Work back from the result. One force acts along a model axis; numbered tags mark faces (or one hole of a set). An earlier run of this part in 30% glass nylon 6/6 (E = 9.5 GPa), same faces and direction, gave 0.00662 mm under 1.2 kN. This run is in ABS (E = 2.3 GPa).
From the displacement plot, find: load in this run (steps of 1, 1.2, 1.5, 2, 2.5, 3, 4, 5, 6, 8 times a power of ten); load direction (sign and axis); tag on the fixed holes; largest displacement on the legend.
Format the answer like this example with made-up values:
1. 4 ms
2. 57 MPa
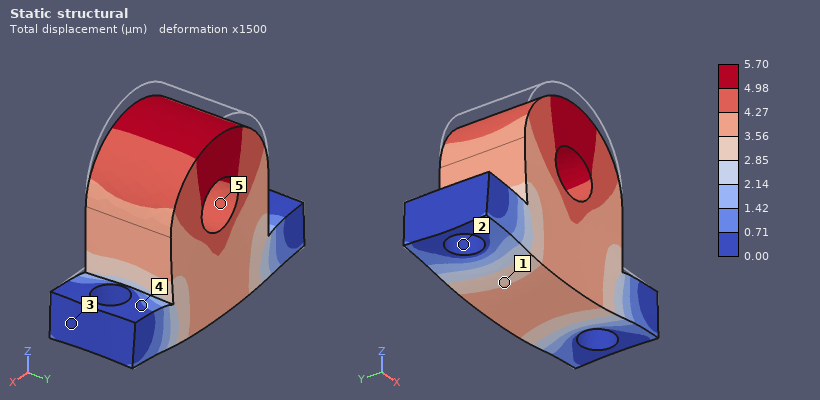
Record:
1. 250 N
2. -Z
3. 2
4. 5.70 µm
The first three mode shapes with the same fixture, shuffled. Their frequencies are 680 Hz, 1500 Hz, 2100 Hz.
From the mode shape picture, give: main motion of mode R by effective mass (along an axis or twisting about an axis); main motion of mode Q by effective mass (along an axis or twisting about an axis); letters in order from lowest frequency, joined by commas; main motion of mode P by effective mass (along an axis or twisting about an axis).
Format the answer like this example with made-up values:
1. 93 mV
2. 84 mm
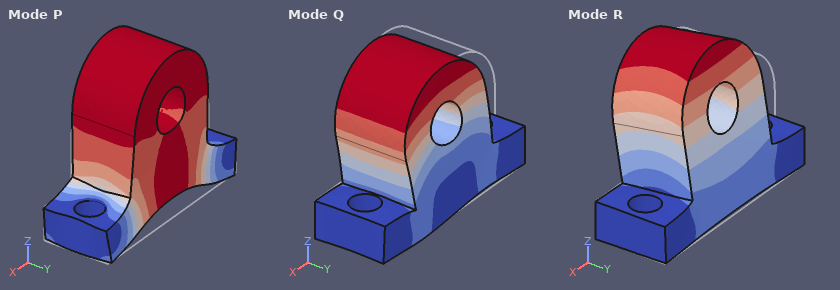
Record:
1. along Y
2. along X
3. R, Q, P
4. along Z
